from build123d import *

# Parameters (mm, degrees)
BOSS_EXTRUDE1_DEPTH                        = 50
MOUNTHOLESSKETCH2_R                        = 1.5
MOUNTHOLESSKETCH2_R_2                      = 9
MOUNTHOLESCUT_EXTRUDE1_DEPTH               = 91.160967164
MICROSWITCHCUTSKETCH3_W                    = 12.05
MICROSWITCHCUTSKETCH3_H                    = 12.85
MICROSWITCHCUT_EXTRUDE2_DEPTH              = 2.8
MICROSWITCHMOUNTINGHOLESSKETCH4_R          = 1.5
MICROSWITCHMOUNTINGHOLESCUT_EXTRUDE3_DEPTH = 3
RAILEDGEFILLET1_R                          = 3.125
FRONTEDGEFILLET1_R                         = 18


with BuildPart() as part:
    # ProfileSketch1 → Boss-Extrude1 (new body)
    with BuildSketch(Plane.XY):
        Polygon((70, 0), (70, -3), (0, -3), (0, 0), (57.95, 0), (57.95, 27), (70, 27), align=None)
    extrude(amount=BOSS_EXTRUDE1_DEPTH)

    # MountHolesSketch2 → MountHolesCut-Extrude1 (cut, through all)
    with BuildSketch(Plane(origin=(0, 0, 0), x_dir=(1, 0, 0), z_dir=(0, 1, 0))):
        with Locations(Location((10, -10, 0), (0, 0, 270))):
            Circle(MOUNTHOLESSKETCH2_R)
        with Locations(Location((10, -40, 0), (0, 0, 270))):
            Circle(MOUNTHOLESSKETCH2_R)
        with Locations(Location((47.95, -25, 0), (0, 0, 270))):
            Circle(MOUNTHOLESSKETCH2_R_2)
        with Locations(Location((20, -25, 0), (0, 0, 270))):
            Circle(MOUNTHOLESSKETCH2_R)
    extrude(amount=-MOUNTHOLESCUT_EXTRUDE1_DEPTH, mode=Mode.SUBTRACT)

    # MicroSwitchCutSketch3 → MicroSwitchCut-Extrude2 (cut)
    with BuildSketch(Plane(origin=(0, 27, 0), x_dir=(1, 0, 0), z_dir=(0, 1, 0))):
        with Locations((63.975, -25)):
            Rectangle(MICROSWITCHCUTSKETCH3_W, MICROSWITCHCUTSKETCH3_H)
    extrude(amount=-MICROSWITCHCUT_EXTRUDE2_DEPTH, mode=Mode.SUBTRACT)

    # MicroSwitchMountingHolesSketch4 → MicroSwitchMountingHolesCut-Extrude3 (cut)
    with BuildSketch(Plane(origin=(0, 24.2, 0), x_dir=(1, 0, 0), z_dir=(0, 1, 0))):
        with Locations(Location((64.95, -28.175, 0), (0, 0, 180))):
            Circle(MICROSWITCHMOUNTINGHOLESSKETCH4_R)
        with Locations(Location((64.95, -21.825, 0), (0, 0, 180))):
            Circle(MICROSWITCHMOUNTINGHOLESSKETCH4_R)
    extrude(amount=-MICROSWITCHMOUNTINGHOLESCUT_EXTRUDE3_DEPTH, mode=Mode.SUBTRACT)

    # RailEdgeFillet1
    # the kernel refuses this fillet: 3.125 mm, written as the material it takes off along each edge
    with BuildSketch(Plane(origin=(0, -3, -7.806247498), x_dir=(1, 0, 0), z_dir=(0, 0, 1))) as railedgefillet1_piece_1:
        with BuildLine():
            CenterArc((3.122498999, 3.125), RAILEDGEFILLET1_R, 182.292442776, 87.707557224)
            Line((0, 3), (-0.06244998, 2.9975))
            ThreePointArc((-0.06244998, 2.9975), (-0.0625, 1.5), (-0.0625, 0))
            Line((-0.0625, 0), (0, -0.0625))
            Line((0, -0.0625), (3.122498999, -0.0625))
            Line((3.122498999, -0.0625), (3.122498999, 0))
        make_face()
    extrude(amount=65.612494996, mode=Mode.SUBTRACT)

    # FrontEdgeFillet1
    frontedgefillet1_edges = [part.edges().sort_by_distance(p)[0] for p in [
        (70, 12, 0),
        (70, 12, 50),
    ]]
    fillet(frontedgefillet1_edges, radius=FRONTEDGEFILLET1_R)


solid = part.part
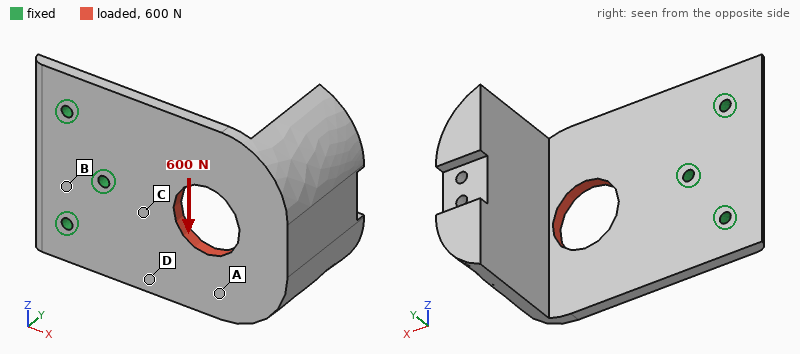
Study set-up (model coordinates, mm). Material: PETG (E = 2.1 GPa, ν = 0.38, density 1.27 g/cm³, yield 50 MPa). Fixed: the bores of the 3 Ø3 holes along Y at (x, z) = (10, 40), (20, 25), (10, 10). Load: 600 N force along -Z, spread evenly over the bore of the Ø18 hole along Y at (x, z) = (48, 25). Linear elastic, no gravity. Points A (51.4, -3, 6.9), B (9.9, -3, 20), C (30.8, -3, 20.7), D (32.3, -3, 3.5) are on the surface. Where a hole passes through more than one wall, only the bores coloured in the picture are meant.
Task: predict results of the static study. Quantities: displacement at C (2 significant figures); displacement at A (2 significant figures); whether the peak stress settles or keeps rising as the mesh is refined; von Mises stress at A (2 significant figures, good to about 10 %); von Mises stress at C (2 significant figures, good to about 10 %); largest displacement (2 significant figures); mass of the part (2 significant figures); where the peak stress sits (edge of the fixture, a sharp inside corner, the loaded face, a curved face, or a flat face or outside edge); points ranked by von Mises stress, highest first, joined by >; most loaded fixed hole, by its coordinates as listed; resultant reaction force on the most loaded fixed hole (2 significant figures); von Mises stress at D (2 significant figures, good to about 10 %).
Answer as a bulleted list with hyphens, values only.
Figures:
- 0.17 mm
- 0.55 mm
- keeps rising
- 4.7 MPa
- 12 MPa
- 0.73 mm
- 27 g
- edge of the fixture
- C > D > A > B
- (20, 25)
- 610 N
- 8.4 MPa
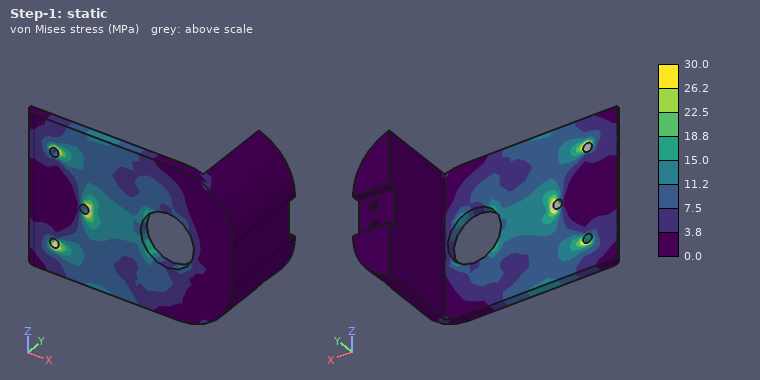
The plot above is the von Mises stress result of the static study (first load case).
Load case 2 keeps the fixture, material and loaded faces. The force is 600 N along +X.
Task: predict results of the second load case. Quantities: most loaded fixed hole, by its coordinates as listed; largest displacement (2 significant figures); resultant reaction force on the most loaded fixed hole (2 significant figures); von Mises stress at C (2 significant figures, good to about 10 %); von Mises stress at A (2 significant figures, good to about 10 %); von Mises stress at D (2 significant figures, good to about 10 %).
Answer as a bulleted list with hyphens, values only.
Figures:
- (20, 25)
- 0.13 mm
- 230 N
- 5.3 MPa
- 2.3 MPa
- 3.0 MPa
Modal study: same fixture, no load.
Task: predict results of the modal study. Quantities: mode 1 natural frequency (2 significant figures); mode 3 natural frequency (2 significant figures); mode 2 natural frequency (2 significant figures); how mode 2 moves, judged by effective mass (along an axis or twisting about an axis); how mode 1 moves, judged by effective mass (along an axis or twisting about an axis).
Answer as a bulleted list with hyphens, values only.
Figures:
- 88 Hz
- 380 Hz
- 200 Hz
- along Z
- along Y
